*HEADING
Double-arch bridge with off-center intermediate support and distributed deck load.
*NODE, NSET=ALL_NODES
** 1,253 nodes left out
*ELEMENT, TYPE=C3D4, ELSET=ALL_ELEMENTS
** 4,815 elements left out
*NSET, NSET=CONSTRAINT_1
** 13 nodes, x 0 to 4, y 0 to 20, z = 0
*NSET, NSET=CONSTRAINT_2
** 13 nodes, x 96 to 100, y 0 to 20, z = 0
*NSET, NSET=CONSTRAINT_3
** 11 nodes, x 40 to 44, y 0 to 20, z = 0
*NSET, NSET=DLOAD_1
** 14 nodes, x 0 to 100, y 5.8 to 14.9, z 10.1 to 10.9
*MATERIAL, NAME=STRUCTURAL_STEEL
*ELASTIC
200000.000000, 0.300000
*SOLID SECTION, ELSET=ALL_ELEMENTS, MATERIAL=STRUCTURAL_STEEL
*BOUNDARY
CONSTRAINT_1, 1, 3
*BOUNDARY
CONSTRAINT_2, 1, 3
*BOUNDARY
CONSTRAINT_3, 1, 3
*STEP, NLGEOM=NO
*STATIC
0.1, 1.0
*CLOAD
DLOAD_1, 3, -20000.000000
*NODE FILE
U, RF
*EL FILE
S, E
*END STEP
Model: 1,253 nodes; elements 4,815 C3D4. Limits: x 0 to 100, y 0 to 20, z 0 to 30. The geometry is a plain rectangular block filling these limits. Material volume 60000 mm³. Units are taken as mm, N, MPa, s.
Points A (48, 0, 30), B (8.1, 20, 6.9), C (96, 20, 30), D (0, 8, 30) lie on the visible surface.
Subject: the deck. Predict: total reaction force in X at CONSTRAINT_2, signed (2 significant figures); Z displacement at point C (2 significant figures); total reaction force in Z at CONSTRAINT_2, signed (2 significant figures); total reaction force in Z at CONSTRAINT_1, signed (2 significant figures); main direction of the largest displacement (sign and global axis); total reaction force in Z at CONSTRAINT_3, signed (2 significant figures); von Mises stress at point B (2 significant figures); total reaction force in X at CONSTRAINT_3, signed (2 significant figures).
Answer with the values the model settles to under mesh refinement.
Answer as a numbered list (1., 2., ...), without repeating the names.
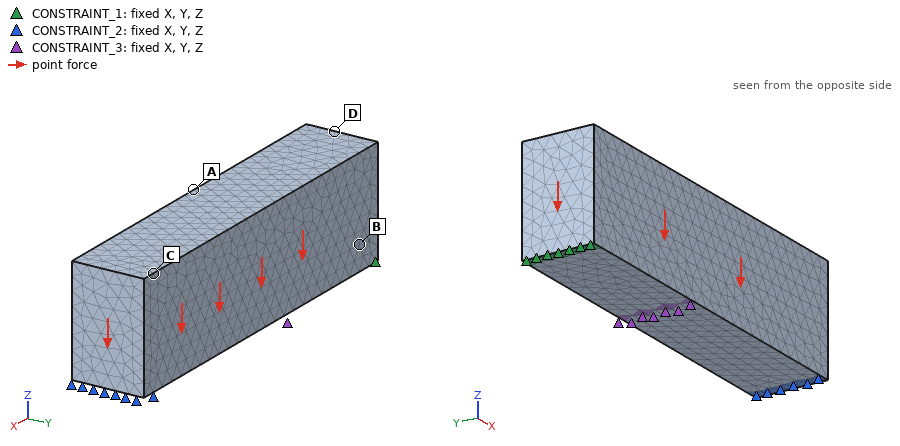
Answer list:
1. -23000 N
2. -0.054 mm
3. 1.0e+05 N
4. 85000 N
5. -Z
6. 91000 N
7. 200 MPa
8. 12000 N
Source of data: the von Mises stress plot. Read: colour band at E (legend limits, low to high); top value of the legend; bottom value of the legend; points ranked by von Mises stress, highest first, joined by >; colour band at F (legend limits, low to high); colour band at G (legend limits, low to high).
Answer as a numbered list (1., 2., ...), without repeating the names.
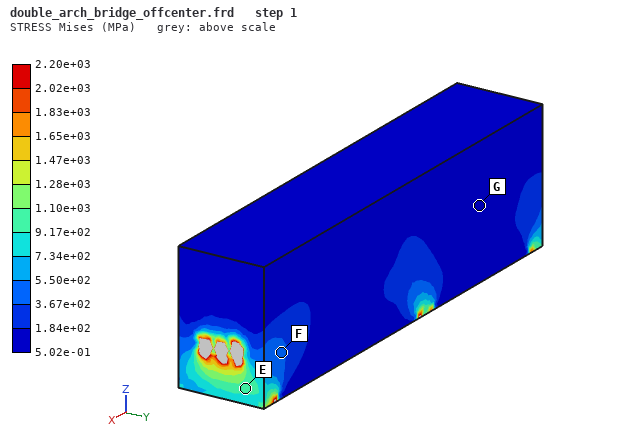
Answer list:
1. 9.17e+02 to 1.10e+03 MPa
2. 2.20e+03 MPa
3. 5.02e-01 MPa
4. E > F > G
5. 3.67e+02 to 5.50e+02 MPa
6. 5.02e-01 to 1.84e+02 MPa
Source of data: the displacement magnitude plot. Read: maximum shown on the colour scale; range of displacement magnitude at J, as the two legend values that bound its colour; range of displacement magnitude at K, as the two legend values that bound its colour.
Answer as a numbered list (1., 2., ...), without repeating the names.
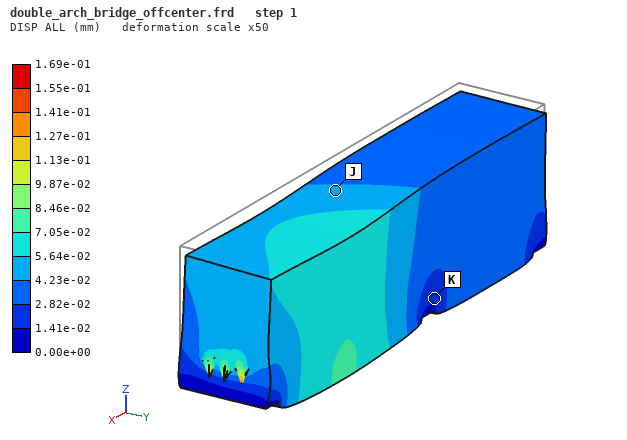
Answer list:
1. 1.69e-01 mm
2. 4.23e-02 to 5.64e-02 mm
3. 1.41e-02 to 2.82e-02 mm
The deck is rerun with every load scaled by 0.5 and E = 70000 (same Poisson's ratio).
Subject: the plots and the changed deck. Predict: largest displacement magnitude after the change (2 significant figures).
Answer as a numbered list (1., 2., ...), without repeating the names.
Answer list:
1. 0.24 mm
